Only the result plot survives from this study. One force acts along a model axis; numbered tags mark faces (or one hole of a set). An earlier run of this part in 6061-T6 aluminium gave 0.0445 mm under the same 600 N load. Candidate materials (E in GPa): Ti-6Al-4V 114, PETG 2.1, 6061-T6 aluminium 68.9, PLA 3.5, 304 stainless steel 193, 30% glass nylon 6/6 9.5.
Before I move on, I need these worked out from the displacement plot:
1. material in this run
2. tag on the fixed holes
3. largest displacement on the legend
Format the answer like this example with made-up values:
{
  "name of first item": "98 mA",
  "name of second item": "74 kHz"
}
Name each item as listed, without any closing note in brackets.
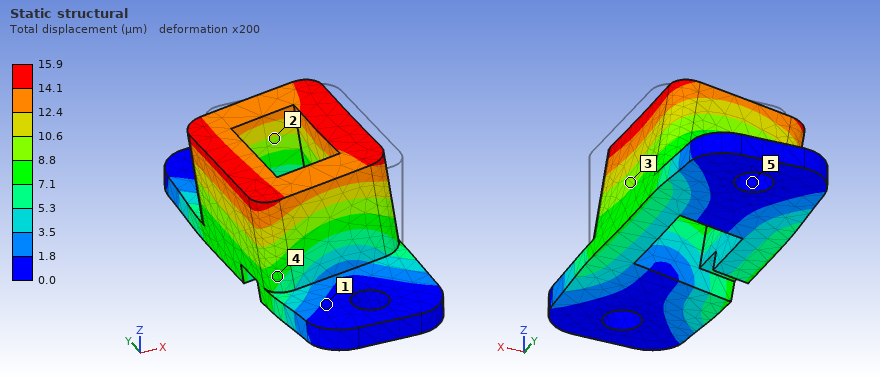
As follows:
{
  "material in this run": "304 stainless steel",
  "tag on the fixed holes": "5",
  "largest displacement on the legend": "15.9 µm"
}
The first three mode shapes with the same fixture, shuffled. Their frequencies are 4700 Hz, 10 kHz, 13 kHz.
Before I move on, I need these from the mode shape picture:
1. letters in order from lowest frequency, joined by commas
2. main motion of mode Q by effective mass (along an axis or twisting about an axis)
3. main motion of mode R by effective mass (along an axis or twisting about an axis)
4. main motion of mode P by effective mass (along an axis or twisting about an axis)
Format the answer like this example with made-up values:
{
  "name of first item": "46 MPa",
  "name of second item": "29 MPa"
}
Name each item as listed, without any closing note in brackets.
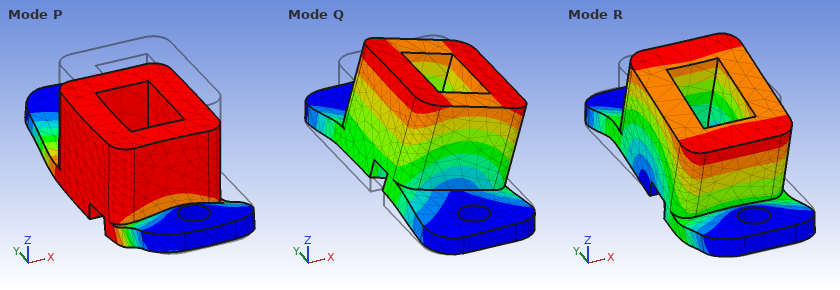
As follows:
{
  "letters in order from lowest frequency, joined by commas": "Q, P, R",
  "main motion of mode Q by effective mass": "along X",
  "main motion of mode R by effective mass": "along Y",
  "main motion of mode P by effective mass": "along Z"
}
